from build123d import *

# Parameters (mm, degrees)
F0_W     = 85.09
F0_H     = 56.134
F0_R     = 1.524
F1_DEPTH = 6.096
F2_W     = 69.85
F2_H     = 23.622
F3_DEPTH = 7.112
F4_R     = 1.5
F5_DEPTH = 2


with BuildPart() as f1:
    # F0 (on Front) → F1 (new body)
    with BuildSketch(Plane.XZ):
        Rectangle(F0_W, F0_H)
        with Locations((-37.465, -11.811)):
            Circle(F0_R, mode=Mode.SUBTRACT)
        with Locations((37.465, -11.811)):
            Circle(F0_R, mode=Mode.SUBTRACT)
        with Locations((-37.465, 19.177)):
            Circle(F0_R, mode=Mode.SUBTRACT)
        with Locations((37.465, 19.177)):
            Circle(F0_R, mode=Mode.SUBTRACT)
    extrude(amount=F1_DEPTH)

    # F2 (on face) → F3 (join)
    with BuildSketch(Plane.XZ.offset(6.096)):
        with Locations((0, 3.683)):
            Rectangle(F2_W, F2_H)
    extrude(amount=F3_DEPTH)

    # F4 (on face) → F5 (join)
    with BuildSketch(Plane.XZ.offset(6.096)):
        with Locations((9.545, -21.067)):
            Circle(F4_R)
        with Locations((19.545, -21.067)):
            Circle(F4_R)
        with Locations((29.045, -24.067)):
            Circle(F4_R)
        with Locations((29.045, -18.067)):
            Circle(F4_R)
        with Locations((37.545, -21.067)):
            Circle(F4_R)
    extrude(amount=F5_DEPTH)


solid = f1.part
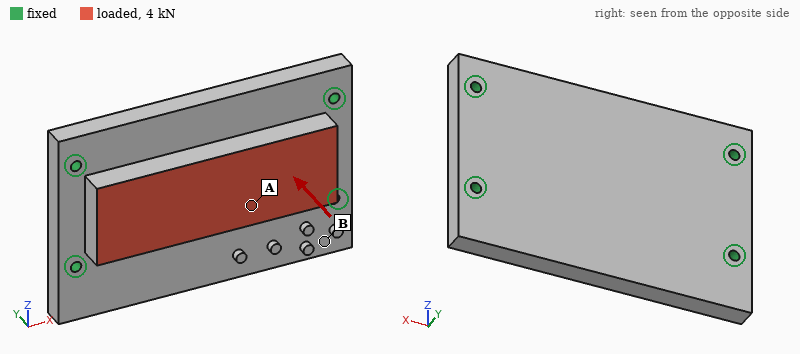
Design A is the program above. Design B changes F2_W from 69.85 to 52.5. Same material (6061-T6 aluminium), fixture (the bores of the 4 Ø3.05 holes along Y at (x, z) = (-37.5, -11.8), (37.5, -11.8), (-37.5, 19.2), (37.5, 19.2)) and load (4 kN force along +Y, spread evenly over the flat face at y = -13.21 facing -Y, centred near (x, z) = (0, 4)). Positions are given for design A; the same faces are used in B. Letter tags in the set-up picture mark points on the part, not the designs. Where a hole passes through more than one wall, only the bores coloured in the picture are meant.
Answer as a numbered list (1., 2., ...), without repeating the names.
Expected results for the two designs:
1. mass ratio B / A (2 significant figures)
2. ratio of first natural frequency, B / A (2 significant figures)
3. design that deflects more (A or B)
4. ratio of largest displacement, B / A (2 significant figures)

1. 0.93
2. 0.95
3. B
4. 1.3
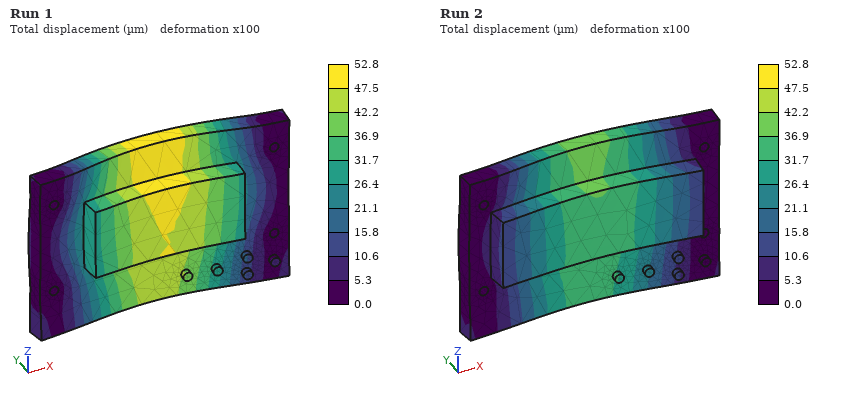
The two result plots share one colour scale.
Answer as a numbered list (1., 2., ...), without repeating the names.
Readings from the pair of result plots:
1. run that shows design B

1. Run 1
